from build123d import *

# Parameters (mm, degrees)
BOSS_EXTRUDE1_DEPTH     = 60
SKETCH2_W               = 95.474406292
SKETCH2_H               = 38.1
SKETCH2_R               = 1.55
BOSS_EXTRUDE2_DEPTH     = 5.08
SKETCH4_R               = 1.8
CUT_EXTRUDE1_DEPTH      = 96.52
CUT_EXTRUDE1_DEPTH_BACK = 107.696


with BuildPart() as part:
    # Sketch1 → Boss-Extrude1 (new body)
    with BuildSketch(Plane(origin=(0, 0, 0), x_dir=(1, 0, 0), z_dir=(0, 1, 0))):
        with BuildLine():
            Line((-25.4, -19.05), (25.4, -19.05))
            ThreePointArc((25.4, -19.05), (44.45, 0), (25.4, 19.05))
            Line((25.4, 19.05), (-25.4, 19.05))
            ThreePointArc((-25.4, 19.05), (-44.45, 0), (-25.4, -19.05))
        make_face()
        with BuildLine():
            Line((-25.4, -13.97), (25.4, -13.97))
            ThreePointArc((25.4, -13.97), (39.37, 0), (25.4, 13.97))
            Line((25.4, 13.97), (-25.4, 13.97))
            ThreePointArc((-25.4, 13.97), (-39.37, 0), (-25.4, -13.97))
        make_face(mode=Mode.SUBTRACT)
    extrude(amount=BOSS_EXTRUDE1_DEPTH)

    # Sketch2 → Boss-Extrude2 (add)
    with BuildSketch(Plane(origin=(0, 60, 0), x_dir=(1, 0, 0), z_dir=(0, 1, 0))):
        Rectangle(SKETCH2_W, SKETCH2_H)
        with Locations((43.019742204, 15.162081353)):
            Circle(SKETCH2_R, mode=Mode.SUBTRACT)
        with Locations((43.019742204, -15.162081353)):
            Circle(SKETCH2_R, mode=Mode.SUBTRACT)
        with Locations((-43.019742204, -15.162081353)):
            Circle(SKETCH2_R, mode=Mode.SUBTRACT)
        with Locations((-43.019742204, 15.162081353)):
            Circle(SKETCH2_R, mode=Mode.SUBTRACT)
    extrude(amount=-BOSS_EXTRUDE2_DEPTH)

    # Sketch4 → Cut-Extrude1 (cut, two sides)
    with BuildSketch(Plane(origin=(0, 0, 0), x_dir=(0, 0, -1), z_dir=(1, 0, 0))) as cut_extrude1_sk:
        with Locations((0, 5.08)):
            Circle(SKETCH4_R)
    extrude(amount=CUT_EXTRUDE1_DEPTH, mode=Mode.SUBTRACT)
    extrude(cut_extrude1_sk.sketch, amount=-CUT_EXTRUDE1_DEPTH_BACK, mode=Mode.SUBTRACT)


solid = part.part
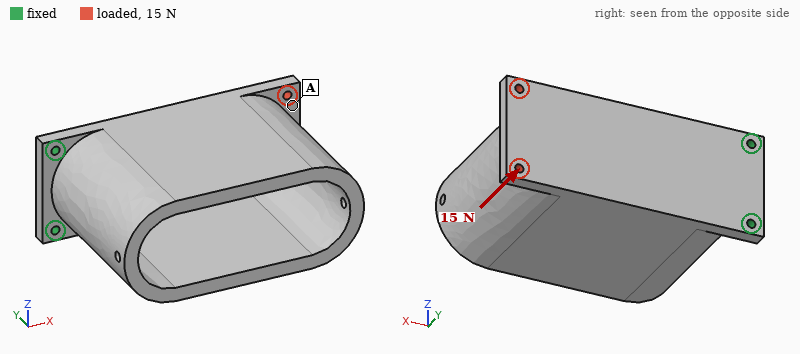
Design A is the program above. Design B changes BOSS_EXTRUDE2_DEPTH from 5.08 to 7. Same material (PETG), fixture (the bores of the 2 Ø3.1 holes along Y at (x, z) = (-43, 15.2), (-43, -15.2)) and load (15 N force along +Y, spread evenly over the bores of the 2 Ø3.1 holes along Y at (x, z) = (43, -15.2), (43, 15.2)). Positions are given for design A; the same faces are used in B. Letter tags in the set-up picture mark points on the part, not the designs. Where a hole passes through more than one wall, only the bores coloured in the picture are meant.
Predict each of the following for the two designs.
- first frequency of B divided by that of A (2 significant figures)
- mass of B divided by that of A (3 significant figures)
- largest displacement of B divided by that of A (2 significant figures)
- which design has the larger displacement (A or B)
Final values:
1.4
1.07
0.50
A
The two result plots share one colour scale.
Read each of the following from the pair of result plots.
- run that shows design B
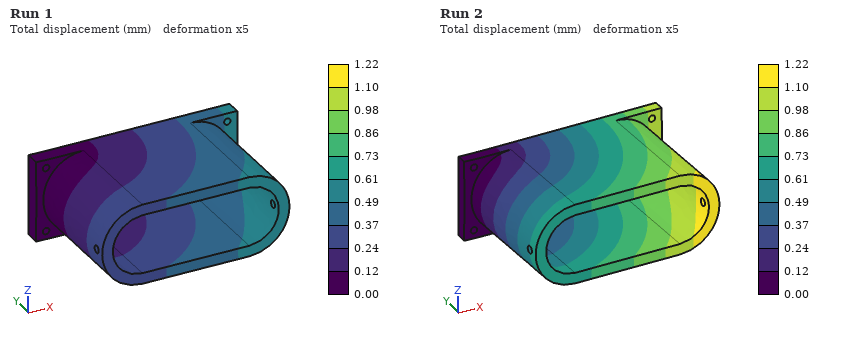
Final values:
Run 1
